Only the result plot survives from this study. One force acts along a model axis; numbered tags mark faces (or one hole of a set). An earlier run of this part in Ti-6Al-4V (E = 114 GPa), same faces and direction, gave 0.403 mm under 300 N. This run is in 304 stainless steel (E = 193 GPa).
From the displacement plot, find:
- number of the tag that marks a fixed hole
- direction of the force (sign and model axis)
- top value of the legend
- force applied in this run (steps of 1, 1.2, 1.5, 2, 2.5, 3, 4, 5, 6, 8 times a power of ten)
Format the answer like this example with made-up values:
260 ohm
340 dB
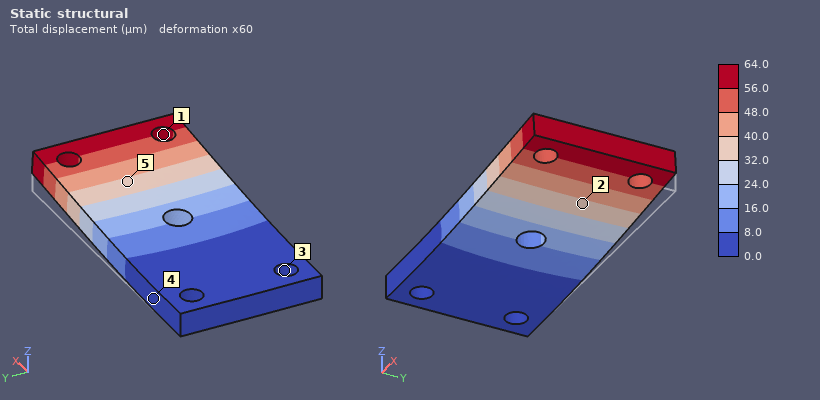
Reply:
3
+Z
64.0 µm
80 N
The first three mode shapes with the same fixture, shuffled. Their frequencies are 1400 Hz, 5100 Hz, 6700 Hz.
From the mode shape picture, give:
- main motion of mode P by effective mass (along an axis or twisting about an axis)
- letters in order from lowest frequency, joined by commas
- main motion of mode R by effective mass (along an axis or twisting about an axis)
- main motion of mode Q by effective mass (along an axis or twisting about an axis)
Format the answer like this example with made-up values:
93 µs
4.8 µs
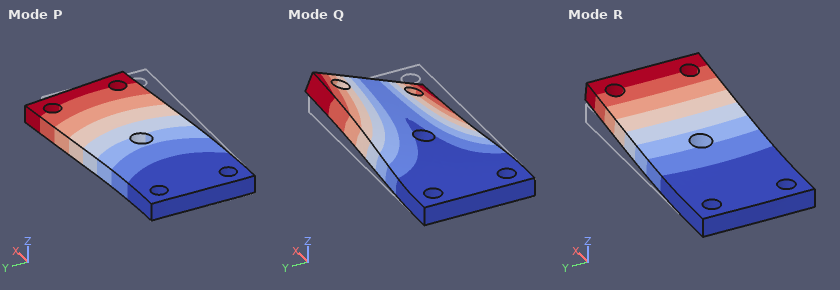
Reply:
along Y
R, Q, P
along Z
twisting about X
